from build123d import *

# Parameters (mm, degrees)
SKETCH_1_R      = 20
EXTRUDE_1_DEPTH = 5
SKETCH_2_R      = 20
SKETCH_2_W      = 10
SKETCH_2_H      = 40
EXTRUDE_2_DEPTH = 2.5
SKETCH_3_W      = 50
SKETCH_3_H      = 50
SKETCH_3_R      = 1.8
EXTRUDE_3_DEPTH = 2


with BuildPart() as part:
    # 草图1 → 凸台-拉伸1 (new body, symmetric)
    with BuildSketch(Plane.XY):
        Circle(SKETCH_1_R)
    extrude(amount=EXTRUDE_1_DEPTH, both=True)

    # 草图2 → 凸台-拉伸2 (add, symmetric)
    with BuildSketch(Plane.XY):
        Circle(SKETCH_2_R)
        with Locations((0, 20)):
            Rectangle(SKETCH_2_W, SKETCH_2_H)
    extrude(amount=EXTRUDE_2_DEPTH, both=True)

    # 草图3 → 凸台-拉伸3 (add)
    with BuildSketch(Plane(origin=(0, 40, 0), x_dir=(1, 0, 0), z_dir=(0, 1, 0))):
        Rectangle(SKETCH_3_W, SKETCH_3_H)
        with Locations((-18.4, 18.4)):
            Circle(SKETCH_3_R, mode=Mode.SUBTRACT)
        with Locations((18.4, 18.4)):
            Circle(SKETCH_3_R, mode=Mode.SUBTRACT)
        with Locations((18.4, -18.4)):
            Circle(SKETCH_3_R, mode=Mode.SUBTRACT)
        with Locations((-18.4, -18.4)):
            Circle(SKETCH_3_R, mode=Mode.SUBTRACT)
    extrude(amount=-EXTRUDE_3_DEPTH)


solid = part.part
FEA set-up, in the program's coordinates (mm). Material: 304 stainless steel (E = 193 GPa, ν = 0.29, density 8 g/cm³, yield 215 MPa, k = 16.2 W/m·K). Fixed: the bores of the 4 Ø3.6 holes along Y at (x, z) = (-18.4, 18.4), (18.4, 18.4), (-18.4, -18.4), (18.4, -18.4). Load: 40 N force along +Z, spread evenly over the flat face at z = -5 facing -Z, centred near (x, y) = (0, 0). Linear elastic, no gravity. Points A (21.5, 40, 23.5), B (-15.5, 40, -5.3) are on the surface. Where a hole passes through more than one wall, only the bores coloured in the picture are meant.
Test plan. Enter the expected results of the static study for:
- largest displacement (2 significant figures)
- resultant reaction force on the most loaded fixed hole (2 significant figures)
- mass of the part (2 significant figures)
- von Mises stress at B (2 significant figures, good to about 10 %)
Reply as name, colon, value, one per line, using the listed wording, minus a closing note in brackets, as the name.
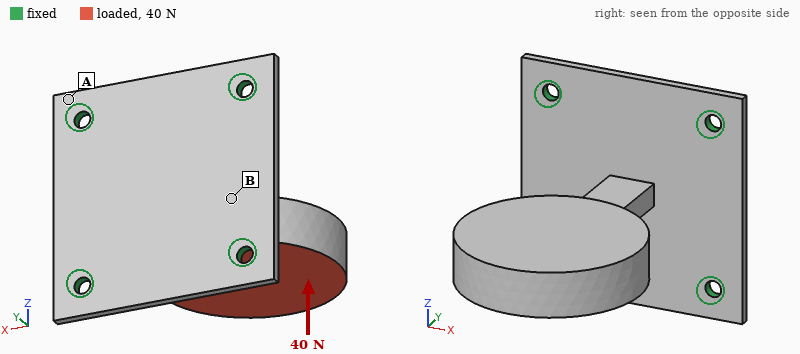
largest displacement: 0.13 mm
resultant reaction force on the most loaded fixed hole: 29 N
mass of the part: 150 g
von Mises stress at B: 10.0 MPa
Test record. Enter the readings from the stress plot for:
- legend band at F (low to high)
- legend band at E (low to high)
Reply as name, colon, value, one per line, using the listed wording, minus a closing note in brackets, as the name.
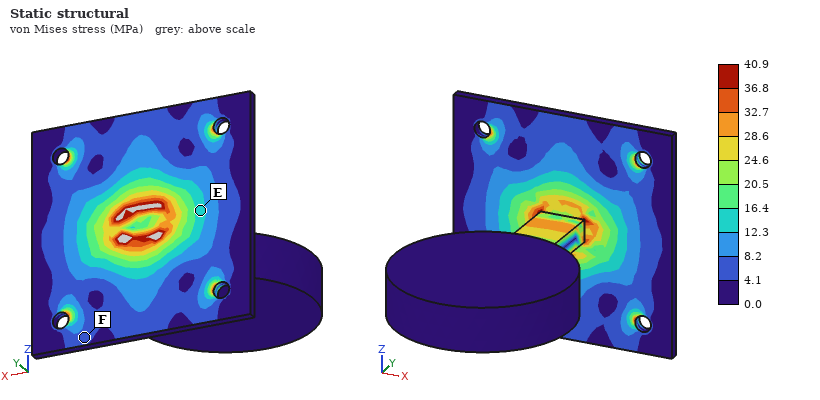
legend band at F: 4.1 to 8.2 MPa
legend band at E: 12.3 to 16.4 MPa
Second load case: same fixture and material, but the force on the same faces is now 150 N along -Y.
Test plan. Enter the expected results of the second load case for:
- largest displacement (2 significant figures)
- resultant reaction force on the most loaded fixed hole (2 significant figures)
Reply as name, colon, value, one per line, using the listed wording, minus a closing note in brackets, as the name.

largest displacement: 74 µm
resultant reaction force on the most loaded fixed hole: 51 N
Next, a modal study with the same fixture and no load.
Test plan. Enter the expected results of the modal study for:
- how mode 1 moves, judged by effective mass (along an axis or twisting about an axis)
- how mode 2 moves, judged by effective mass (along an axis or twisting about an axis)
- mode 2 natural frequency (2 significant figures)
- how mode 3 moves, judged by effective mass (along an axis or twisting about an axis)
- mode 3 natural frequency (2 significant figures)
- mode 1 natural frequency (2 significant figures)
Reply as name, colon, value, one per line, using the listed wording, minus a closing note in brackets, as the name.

how mode 1 moves, judged by effective mass: along Z
how mode 2 moves, judged by effective mass: along X
mode 2 natural frequency: 440 Hz
how mode 3 moves, judged by effective mass: along Y
mode 3 natural frequency: 1500 Hz
mode 1 natural frequency: 340 Hz
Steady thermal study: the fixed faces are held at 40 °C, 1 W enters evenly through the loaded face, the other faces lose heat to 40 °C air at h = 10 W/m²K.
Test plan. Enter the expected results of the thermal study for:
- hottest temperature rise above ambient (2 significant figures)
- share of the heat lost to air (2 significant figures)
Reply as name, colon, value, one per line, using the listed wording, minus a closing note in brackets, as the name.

hottest temperature rise above ambient: 20 K
share of the heat lost to air: 61 %
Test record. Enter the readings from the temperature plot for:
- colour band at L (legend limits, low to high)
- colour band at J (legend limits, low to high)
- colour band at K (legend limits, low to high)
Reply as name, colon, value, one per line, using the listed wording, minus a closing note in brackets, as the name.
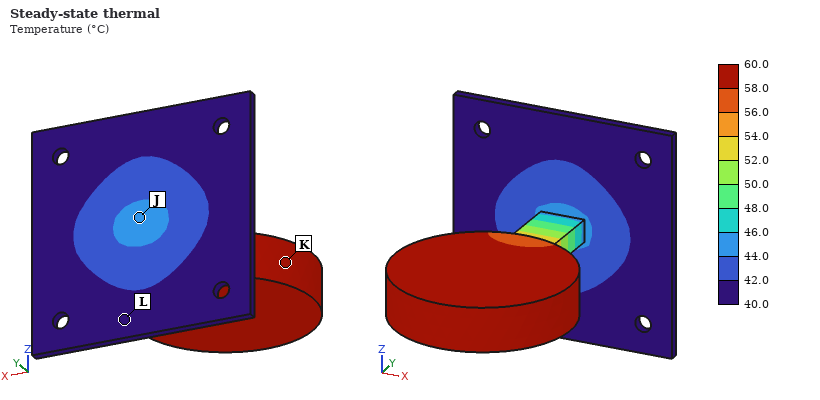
colour band at L: 40.0 to 42.0 °C
colour band at J: 44.0 to 46.0 °C
colour band at K: 58.0 to 60.0 °C
